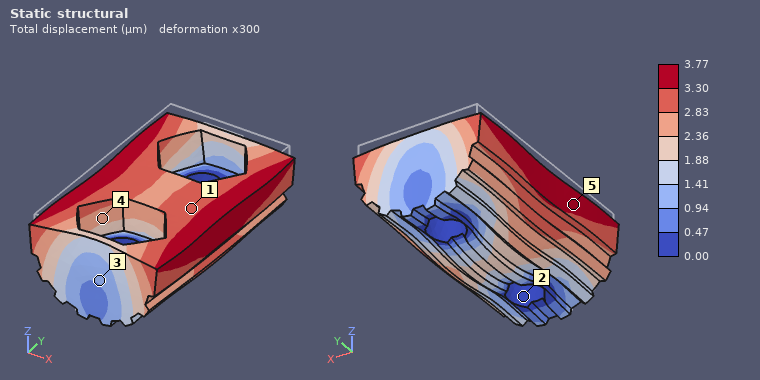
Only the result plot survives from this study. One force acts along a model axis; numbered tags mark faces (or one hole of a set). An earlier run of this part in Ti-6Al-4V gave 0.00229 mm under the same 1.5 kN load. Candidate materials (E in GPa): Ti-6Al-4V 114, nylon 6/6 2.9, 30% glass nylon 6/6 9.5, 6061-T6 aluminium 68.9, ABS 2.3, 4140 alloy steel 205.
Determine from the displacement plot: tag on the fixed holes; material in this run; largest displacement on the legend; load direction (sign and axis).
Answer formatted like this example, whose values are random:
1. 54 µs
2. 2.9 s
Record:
1. 2
2. 6061-T6 aluminium
3. 3.77 µm
4. -Z
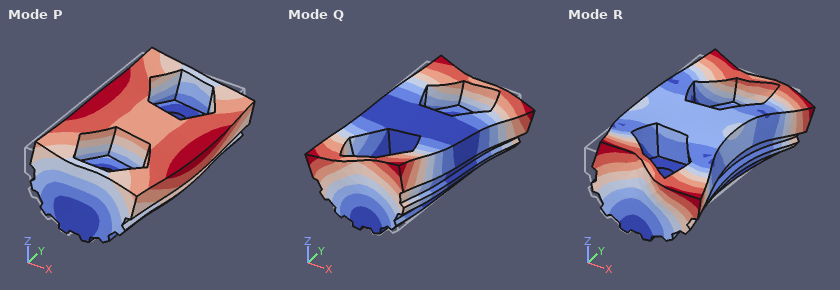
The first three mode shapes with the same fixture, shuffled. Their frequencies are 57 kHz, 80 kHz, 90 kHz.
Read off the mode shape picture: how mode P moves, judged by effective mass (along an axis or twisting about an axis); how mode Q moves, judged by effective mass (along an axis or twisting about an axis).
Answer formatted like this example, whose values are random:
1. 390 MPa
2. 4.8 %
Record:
1. along X
2. twisting about Z
